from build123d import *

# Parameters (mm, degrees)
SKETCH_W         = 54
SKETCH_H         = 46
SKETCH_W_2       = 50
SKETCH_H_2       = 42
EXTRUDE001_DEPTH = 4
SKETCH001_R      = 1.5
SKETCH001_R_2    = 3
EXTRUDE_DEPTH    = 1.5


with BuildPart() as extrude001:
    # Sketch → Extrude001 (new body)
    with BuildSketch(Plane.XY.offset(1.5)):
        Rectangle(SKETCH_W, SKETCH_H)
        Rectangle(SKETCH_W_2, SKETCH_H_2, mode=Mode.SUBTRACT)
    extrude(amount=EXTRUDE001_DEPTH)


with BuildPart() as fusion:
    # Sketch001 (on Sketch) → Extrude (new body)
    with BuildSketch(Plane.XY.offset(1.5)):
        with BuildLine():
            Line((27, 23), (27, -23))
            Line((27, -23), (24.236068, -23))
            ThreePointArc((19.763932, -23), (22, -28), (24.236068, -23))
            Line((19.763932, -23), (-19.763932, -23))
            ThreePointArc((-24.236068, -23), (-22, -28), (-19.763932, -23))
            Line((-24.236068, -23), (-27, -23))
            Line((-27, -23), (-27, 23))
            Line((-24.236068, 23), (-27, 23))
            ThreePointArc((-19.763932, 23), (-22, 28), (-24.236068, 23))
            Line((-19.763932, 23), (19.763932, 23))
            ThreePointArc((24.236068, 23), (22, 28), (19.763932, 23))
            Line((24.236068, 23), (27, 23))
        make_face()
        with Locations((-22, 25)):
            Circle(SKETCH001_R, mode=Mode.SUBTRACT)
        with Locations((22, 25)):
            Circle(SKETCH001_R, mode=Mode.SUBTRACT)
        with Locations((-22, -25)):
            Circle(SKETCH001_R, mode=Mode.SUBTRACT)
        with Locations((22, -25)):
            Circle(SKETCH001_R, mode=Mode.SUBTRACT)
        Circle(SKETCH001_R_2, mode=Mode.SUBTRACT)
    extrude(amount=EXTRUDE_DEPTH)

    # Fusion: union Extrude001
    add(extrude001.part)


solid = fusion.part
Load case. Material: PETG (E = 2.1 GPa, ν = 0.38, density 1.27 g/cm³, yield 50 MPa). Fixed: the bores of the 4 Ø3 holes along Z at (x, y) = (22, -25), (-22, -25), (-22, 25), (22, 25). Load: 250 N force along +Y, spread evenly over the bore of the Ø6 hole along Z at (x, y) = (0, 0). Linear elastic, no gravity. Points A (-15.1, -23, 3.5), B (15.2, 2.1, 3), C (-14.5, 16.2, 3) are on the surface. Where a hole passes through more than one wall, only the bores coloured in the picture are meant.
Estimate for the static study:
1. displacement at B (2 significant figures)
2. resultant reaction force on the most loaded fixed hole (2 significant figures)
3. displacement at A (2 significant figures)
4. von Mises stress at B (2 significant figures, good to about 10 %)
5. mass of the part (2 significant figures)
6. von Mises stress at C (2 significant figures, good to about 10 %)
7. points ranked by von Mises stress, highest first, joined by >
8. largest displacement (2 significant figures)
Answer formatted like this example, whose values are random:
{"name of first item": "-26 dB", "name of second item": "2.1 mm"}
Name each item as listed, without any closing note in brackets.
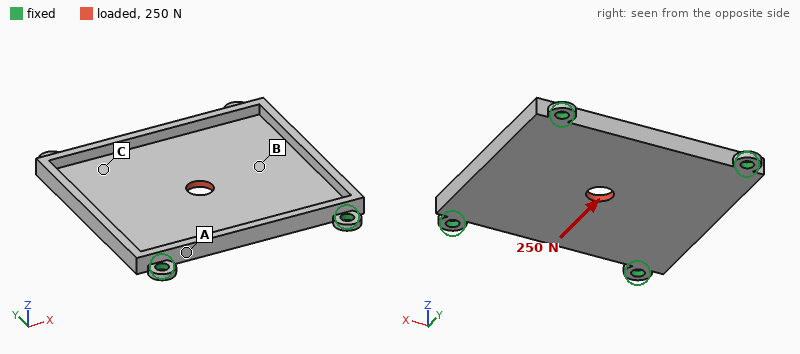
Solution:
{"displacement at B": "41 µm", "resultant reaction force on the most loaded fixed hole": "68 N", "displacement at A": "35 µm", "von Mises stress at B": "2.8 MPa", "mass of the part": "6.0 g", "von Mises stress at C": "4.5 MPa", "points ranked by von Mises stress, highest first, joined by >": "C > B > A", "largest displacement": "96 µm"}
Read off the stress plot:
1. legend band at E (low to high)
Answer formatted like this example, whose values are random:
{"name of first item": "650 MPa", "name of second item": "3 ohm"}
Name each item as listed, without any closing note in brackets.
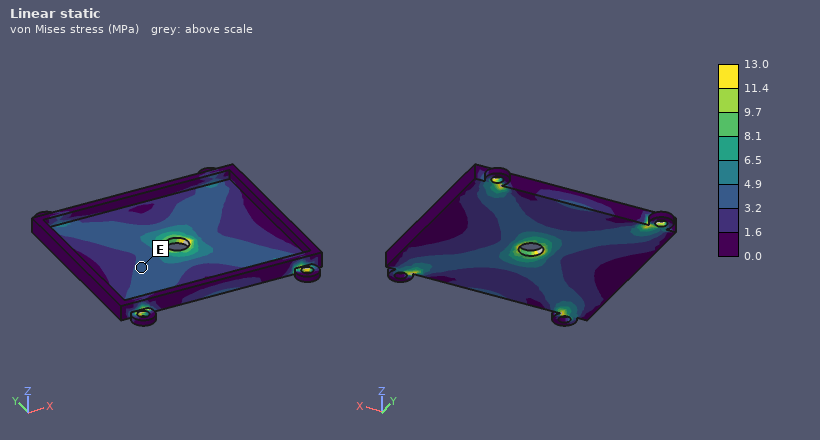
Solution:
{"legend band at E": "3.2 to 4.9 MPa"}
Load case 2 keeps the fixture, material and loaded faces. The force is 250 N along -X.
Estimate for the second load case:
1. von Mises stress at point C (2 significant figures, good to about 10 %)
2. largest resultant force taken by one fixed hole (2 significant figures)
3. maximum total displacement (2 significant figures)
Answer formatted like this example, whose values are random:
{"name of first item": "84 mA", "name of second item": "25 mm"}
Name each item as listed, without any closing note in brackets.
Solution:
{"von Mises stress at point C": "4.7 MPa", "largest resultant force taken by one fixed hole": "68 N", "maximum total displacement": "0.12 mm"}
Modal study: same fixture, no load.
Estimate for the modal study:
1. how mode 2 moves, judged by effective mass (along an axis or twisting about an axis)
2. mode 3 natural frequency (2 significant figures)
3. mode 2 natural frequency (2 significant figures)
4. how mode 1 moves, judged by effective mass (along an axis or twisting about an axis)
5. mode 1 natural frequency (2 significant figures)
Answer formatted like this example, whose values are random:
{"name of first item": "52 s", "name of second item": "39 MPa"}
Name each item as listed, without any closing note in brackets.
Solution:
{"how mode 2 moves, judged by effective mass": "twisting about Y", "mode 3 natural frequency": "1500 Hz", "mode 2 natural frequency": "1200 Hz", "how mode 1 moves, judged by effective mass": "along Z", "mode 1 natural frequency": "730 Hz"}
